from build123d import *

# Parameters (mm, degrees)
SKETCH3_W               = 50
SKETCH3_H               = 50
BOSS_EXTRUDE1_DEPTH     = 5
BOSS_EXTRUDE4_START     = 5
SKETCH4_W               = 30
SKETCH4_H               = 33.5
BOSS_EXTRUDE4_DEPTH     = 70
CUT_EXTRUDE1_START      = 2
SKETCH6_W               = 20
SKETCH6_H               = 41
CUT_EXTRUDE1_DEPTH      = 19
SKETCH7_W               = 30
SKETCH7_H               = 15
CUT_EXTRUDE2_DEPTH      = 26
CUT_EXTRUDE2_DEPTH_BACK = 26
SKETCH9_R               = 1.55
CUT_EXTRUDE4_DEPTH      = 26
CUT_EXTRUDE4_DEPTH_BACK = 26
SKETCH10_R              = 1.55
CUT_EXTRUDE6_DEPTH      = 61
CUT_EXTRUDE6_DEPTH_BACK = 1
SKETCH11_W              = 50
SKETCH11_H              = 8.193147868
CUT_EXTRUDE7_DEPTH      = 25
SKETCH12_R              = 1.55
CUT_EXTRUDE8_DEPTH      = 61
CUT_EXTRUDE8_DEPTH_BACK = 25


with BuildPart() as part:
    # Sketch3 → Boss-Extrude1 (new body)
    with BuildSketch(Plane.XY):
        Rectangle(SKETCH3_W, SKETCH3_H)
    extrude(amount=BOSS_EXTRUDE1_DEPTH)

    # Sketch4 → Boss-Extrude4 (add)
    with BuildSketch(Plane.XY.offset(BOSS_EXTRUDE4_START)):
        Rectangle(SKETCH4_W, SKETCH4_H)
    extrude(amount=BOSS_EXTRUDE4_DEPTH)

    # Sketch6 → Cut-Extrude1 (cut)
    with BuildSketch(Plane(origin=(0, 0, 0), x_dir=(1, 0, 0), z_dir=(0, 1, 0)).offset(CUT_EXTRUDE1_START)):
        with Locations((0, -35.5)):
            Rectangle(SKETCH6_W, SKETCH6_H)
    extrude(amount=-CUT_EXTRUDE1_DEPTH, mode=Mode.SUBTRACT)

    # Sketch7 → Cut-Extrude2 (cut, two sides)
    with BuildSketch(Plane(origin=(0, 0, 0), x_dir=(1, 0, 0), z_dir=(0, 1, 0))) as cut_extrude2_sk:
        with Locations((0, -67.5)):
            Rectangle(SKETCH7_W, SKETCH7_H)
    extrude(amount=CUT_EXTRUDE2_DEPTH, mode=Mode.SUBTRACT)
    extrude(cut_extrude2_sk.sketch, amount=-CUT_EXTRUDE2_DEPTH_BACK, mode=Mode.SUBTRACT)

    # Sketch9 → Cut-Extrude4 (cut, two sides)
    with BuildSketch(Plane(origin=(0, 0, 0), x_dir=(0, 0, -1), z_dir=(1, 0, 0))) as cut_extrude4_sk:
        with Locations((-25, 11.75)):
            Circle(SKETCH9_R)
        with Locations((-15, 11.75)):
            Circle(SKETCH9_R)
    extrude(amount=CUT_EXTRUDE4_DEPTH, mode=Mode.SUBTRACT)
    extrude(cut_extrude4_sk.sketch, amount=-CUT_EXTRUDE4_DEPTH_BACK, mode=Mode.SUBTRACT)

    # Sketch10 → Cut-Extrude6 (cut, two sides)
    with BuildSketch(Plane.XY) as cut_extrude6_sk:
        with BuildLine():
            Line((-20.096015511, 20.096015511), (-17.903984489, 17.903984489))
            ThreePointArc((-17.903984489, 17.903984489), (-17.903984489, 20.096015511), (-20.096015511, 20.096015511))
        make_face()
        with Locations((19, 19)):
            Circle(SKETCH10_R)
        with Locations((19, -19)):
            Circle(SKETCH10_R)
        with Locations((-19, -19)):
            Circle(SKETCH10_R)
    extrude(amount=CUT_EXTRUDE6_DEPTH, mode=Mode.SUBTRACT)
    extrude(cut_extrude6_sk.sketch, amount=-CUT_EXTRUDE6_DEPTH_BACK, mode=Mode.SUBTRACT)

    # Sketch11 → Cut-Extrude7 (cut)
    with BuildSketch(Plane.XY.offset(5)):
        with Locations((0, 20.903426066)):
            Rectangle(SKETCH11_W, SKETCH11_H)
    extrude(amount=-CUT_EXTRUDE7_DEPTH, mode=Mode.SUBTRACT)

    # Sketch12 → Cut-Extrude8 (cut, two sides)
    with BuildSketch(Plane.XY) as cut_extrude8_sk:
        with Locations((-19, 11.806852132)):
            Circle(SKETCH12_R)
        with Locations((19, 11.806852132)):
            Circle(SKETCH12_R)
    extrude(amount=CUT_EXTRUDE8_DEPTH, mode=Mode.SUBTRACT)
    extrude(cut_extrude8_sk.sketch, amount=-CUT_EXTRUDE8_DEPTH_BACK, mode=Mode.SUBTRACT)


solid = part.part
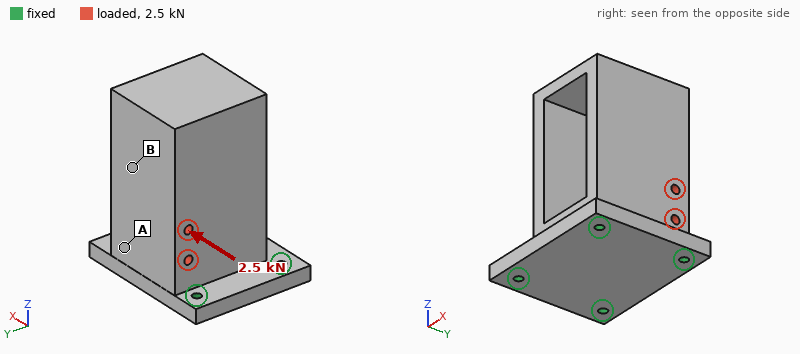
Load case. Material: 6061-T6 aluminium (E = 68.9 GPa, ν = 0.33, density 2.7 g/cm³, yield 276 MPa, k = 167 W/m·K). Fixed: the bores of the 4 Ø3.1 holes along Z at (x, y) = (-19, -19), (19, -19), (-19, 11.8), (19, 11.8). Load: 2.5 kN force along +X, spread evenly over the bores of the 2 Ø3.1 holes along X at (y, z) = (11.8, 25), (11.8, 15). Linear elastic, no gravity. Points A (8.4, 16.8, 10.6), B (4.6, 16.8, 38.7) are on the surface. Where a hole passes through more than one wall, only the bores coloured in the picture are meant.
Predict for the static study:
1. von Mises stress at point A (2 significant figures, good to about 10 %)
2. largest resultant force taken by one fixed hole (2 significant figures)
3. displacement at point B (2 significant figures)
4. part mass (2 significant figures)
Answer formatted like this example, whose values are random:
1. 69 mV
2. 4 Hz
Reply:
1. 16 MPa
2. 1.3 kN
3. 19 µm
4. 130 g
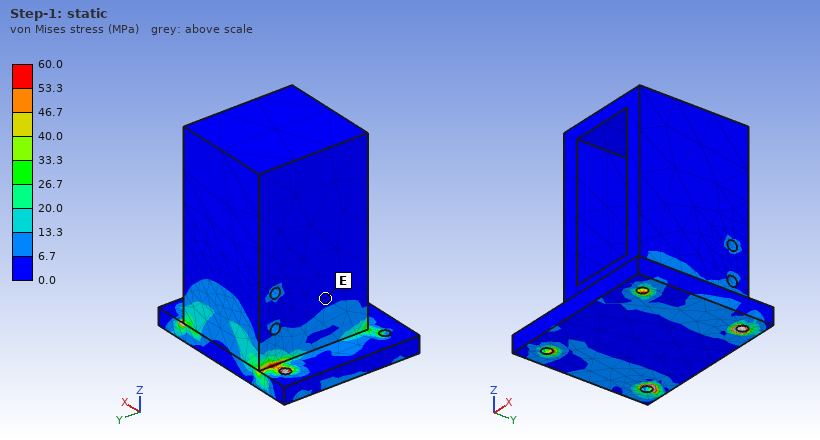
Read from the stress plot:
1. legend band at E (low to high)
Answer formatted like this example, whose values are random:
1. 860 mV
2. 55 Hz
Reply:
1. 0.0 to 6.7 MPa
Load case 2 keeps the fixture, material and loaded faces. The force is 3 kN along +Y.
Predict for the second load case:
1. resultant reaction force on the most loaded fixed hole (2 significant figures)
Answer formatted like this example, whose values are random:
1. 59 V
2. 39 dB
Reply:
1. 1.3 kN
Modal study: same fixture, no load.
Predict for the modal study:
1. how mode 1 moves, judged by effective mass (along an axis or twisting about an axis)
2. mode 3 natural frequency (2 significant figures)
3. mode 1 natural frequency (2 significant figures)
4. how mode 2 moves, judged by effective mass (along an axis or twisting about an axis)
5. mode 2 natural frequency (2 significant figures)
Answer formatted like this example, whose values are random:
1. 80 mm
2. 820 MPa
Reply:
1. along Y
2. 8300 Hz
3. 3500 Hz
4. along X
5. 3700 Hz
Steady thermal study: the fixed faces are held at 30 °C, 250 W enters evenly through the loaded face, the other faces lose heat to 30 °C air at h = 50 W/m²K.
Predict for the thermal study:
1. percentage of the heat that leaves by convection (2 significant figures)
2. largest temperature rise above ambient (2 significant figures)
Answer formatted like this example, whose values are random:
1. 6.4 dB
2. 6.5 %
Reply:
1. 14 %
2. 79 K
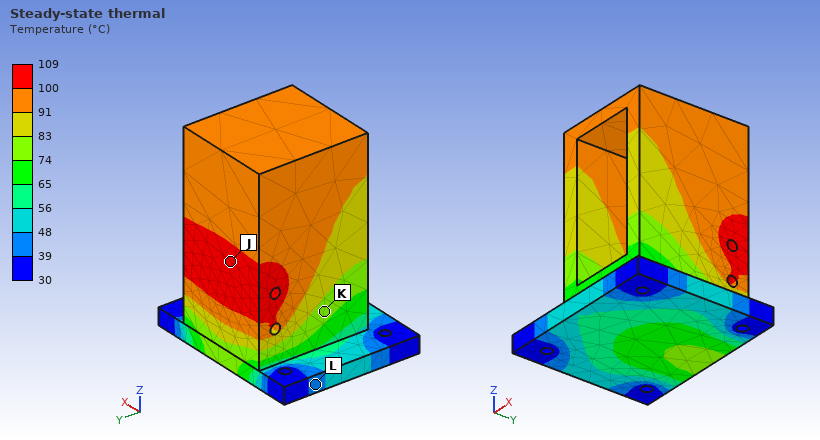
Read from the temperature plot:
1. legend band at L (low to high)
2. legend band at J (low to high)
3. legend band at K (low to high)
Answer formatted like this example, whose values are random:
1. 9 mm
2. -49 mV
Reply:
1. 39 to 48 °C
2. 100 to 109 °C
3. 74 to 83 °C
